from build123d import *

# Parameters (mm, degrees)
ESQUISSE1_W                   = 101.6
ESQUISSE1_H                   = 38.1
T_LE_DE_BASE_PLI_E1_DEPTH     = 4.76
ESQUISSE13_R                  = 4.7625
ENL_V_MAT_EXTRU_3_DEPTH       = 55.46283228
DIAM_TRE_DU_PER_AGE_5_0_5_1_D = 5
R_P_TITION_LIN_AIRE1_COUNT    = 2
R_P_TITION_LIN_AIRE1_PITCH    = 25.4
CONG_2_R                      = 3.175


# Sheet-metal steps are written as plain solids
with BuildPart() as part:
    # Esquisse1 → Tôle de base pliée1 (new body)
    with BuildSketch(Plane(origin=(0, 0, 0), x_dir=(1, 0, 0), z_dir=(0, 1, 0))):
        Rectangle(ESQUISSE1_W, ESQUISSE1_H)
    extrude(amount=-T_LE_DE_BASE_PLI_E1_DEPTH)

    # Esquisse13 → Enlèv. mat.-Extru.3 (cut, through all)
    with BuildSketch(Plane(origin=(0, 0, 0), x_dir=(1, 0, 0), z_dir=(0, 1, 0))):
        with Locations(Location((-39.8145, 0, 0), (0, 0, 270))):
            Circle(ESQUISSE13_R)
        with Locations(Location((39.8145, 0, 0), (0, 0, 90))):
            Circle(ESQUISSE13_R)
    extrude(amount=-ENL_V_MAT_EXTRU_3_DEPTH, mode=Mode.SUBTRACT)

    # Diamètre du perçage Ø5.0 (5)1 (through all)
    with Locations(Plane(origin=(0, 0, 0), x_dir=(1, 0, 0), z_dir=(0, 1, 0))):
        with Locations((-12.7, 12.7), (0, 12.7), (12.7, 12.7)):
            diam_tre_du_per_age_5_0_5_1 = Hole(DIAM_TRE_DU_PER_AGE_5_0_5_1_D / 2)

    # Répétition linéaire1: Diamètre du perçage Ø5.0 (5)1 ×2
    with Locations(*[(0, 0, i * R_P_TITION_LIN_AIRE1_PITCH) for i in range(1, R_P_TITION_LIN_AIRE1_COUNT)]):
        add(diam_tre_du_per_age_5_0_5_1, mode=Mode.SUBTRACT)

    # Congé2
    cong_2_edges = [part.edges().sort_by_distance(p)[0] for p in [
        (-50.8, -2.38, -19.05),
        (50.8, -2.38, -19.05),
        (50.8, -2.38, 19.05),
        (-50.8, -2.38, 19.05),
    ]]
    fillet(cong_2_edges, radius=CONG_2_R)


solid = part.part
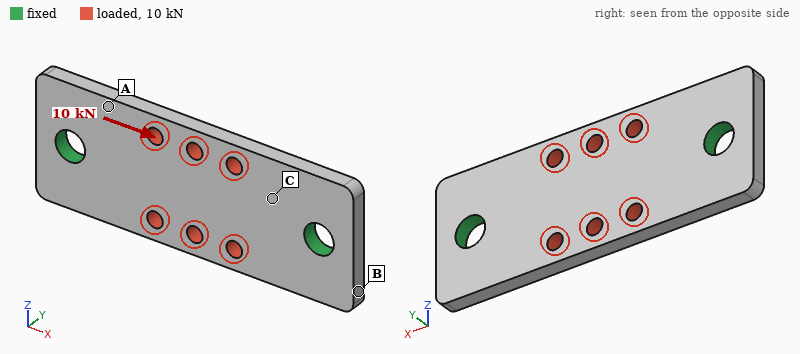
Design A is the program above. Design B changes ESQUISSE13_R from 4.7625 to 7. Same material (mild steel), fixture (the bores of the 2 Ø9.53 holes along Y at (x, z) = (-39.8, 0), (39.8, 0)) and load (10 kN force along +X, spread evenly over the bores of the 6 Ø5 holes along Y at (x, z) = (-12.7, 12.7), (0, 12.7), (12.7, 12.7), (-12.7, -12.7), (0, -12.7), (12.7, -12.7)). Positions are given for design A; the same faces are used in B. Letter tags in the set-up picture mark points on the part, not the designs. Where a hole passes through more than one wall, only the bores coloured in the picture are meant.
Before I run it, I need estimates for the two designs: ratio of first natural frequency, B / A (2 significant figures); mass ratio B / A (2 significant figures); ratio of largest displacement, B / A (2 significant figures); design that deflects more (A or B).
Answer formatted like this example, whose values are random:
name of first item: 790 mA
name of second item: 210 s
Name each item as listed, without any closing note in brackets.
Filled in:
ratio of first natural frequency, B / A: 1.2
mass ratio B / A: 0.95
ratio of largest displacement, B / A: 0.88
design that deflects more: A
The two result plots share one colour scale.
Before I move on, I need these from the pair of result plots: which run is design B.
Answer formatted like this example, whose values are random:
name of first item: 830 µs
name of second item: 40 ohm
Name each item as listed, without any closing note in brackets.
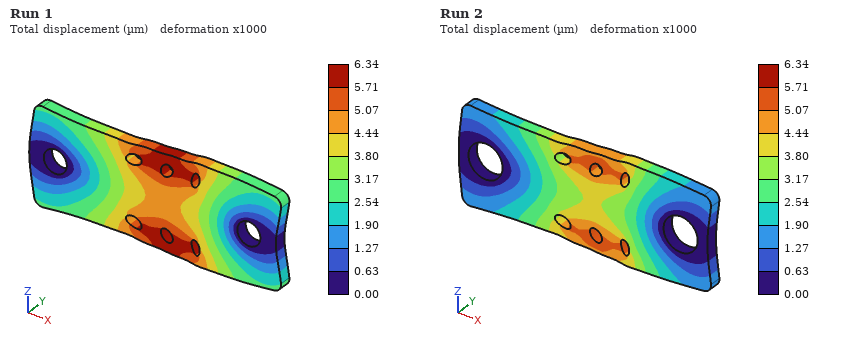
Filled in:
which run is design B: Run 2
